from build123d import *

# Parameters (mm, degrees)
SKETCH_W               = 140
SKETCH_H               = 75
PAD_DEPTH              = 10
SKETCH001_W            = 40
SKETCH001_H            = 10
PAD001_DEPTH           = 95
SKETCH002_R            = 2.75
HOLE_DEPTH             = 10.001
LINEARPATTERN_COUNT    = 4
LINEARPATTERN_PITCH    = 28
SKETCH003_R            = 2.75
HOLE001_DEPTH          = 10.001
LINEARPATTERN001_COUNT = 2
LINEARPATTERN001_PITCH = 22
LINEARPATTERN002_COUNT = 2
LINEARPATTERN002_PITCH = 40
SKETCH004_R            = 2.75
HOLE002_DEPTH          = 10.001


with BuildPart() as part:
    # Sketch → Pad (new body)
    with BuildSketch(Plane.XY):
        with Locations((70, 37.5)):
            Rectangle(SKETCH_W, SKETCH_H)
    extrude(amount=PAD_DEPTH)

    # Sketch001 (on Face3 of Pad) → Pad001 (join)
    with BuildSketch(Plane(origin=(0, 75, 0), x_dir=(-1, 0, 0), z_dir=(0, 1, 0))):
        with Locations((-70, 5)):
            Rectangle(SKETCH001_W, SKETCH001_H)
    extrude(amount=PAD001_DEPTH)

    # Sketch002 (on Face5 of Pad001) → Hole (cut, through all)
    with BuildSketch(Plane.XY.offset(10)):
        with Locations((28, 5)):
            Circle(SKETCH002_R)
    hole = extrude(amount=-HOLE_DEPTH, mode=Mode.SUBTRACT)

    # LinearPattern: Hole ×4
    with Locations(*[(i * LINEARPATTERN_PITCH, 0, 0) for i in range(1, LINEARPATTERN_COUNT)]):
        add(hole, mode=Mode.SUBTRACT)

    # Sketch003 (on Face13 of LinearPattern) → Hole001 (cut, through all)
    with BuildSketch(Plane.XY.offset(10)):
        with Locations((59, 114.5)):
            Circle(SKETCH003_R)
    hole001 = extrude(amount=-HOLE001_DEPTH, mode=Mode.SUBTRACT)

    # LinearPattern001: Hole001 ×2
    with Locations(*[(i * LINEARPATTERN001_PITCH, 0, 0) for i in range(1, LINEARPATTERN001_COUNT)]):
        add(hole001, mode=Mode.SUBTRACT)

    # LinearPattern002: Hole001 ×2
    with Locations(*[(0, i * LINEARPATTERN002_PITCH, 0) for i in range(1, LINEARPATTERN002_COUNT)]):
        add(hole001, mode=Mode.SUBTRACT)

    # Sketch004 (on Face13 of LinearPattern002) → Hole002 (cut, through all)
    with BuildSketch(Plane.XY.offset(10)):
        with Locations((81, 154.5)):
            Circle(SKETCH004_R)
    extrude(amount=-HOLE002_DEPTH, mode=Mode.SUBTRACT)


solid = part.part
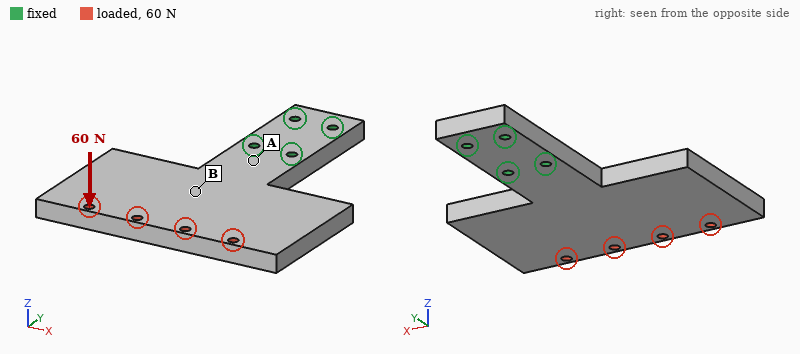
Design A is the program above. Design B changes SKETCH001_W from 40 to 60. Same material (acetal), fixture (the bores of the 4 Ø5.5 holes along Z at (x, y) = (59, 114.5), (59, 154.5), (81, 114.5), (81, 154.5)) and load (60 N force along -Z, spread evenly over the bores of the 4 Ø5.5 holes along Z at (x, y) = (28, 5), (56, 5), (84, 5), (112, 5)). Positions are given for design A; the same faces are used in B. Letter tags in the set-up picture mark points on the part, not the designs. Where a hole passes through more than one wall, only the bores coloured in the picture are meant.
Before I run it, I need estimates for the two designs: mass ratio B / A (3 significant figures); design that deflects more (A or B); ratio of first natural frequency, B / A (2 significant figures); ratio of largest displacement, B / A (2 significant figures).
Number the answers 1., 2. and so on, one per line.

1. 1.13
2. A
3. 1.2
4. 0.70
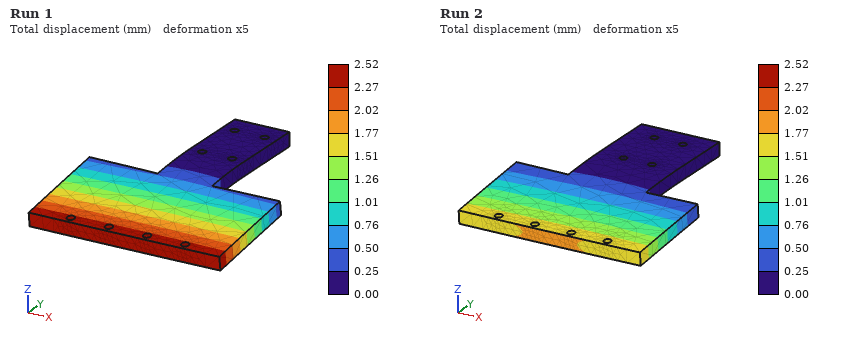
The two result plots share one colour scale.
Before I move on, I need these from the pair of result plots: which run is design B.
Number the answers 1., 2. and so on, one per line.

1. Run 2
